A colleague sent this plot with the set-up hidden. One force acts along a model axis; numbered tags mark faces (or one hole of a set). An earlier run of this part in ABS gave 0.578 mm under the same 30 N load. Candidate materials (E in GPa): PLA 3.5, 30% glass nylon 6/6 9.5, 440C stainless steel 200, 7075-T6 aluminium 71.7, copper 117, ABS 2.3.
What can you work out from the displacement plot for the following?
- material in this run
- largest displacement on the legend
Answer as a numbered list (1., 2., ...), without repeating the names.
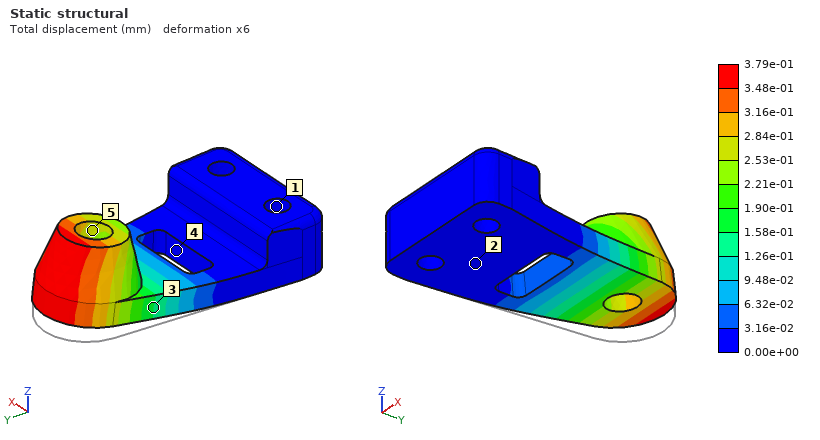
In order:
1. PLA
2. 3.79e-01 mm
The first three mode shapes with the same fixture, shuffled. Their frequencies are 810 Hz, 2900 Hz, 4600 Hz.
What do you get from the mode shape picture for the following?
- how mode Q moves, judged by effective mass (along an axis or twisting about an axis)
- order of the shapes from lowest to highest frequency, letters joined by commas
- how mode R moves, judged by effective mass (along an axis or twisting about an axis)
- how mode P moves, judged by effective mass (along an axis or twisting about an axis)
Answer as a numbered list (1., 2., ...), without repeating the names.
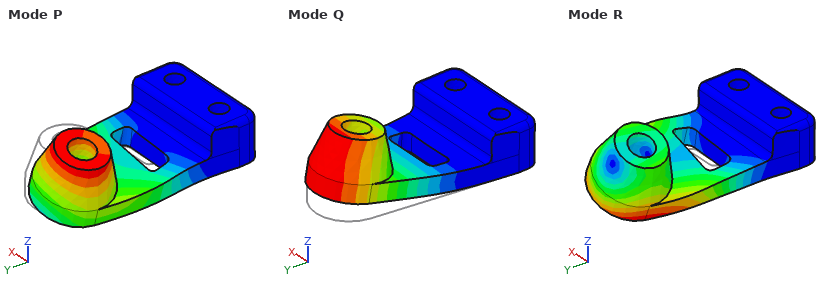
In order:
1. along Z
2. Q, P, R
3. along X
4. along X
